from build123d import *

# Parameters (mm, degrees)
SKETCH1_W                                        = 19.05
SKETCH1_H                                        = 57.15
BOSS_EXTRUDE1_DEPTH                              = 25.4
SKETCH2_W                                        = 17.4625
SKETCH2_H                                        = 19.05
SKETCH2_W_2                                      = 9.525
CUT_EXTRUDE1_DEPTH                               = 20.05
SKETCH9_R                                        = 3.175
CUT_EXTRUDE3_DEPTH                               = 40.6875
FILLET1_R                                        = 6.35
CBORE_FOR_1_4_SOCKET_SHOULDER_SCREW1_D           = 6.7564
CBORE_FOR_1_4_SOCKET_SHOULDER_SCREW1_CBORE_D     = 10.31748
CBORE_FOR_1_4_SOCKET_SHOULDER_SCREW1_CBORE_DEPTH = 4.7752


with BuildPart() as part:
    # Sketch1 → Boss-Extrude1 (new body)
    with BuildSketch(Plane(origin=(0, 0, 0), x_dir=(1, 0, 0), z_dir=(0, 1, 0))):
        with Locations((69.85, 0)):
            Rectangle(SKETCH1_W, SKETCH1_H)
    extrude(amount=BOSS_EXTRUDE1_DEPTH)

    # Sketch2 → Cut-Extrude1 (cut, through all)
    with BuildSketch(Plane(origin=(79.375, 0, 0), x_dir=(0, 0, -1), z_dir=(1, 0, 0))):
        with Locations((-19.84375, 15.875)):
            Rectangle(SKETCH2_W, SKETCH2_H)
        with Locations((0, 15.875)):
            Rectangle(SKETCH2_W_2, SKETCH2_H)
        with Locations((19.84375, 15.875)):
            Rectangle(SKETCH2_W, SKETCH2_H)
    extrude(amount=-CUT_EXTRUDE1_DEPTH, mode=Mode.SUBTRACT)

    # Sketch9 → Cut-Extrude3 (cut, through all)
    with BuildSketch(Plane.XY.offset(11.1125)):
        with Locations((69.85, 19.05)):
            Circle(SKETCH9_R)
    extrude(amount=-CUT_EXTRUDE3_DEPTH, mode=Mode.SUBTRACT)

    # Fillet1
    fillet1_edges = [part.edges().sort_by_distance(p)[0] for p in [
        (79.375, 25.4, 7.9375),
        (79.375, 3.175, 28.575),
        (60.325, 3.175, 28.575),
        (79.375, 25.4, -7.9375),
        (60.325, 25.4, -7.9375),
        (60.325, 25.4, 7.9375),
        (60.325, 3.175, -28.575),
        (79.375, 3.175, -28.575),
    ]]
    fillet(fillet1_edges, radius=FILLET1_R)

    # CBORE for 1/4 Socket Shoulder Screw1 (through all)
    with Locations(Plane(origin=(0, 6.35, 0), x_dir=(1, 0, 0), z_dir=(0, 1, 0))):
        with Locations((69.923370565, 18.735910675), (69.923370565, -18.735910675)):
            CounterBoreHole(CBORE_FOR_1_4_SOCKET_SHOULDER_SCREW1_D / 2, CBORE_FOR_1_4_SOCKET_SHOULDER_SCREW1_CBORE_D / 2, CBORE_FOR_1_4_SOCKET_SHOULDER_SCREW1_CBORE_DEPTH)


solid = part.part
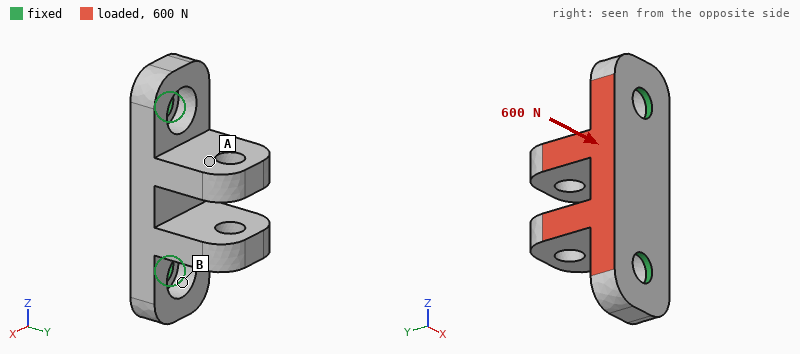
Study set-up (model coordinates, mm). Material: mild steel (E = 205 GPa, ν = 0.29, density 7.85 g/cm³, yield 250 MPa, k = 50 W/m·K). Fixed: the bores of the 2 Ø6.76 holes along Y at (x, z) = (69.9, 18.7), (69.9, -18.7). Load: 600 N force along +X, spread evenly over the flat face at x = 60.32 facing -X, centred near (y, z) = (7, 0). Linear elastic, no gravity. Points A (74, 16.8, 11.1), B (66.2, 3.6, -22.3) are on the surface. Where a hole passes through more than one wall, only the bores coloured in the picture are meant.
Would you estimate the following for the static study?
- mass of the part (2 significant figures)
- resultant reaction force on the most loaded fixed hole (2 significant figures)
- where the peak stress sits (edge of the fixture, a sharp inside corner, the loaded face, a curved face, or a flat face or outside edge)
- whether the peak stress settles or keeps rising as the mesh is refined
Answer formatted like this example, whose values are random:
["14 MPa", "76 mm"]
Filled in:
["77 g", "300 N", "edge of the fixture", "keeps rising"]
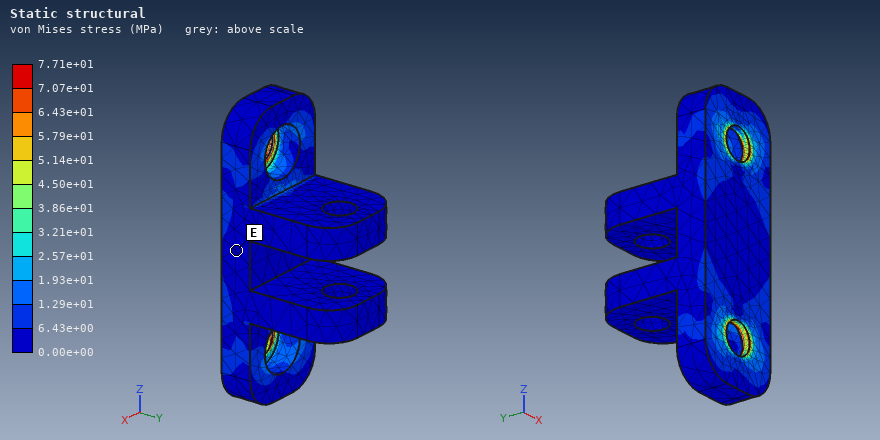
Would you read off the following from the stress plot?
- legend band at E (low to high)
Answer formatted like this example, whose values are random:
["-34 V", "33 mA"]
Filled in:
["0.00e+00 to 6.43e+00 MPa"]
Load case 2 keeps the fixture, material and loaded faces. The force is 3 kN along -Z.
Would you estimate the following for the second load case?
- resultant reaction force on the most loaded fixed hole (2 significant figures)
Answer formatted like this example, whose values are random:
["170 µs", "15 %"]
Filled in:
["1.7 kN"]
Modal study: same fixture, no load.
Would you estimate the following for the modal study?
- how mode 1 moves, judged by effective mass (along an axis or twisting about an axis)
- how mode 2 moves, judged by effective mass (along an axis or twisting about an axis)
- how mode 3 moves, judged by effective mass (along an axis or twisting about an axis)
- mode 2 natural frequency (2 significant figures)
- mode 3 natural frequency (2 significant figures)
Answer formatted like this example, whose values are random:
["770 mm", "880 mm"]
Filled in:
["along X", "along Y", "along Z", "8100 Hz", "11 kHz"]
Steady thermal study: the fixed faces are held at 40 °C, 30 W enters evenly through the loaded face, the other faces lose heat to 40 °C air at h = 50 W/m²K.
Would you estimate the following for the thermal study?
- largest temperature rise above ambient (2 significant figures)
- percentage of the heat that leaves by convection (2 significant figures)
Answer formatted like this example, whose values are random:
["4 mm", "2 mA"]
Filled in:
["41 K", "19 %"]
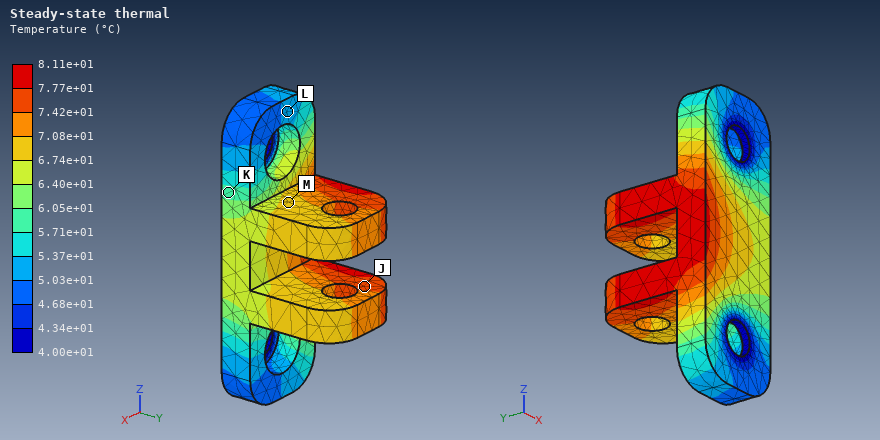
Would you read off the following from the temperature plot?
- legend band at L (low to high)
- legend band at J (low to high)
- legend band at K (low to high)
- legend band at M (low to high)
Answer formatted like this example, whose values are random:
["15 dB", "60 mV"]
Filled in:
["5.03e+01 to 5.37e+01 °C", "7.42e+01 to 7.77e+01 °C", "5.71e+01 to 6.05e+01 °C", "6.74e+01 to 7.08e+01 °C"]
